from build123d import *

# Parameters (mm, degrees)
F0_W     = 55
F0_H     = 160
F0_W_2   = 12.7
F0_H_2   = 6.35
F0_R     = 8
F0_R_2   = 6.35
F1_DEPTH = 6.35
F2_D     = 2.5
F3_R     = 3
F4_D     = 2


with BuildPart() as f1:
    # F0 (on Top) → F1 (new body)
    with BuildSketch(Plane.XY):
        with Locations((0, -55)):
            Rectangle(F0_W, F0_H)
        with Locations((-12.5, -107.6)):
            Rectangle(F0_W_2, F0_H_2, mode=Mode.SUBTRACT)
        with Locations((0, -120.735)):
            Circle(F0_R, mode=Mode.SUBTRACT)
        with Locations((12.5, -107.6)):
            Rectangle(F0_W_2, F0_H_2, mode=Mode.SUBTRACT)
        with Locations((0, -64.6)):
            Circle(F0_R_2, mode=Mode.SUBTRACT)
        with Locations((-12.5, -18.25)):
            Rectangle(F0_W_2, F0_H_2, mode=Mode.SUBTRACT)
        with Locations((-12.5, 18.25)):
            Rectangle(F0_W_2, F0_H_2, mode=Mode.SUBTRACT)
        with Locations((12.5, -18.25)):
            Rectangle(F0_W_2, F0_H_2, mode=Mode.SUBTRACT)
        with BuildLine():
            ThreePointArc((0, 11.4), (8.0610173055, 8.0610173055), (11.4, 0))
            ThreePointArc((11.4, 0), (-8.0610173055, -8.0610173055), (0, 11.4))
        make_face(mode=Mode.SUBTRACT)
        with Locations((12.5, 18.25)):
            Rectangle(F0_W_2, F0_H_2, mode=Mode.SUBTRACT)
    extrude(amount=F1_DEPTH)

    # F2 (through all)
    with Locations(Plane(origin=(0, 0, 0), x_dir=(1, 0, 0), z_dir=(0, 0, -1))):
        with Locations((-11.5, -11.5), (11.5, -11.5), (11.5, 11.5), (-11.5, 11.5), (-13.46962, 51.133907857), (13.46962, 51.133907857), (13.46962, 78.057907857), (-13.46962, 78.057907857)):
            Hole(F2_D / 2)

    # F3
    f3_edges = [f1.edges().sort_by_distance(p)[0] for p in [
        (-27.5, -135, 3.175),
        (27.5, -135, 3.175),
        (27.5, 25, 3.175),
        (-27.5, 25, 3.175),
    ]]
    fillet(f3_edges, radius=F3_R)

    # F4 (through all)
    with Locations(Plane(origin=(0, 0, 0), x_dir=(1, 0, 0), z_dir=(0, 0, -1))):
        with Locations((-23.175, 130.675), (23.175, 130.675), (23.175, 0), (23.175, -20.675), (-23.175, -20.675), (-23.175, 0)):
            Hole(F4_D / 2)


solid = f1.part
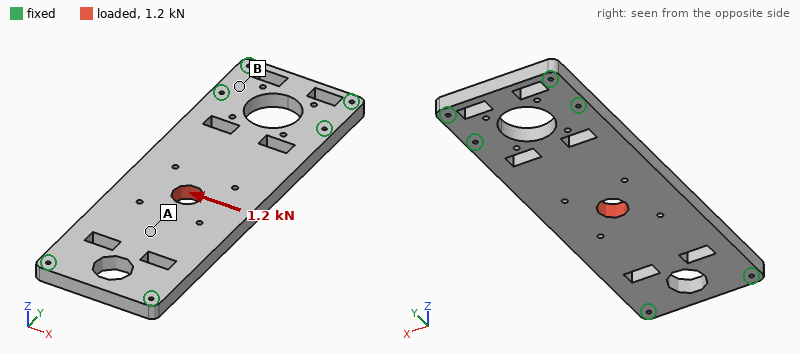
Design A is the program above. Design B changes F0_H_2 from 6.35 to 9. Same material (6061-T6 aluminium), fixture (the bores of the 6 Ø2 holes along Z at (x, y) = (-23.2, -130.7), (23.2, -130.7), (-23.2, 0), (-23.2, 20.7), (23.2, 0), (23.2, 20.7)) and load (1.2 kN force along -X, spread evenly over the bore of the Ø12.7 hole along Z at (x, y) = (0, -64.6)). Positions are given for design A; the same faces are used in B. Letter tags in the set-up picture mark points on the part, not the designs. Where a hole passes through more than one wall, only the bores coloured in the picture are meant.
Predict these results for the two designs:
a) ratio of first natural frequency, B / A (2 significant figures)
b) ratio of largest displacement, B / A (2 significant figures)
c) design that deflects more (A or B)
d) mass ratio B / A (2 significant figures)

1.00
1.1
B
0.97
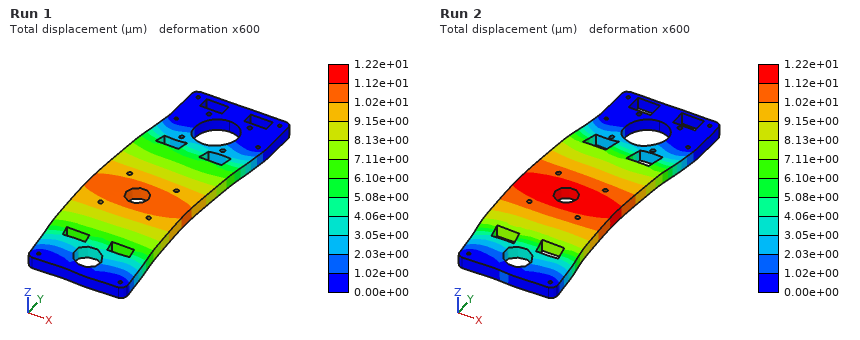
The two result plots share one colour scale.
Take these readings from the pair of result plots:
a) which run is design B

Run 2
